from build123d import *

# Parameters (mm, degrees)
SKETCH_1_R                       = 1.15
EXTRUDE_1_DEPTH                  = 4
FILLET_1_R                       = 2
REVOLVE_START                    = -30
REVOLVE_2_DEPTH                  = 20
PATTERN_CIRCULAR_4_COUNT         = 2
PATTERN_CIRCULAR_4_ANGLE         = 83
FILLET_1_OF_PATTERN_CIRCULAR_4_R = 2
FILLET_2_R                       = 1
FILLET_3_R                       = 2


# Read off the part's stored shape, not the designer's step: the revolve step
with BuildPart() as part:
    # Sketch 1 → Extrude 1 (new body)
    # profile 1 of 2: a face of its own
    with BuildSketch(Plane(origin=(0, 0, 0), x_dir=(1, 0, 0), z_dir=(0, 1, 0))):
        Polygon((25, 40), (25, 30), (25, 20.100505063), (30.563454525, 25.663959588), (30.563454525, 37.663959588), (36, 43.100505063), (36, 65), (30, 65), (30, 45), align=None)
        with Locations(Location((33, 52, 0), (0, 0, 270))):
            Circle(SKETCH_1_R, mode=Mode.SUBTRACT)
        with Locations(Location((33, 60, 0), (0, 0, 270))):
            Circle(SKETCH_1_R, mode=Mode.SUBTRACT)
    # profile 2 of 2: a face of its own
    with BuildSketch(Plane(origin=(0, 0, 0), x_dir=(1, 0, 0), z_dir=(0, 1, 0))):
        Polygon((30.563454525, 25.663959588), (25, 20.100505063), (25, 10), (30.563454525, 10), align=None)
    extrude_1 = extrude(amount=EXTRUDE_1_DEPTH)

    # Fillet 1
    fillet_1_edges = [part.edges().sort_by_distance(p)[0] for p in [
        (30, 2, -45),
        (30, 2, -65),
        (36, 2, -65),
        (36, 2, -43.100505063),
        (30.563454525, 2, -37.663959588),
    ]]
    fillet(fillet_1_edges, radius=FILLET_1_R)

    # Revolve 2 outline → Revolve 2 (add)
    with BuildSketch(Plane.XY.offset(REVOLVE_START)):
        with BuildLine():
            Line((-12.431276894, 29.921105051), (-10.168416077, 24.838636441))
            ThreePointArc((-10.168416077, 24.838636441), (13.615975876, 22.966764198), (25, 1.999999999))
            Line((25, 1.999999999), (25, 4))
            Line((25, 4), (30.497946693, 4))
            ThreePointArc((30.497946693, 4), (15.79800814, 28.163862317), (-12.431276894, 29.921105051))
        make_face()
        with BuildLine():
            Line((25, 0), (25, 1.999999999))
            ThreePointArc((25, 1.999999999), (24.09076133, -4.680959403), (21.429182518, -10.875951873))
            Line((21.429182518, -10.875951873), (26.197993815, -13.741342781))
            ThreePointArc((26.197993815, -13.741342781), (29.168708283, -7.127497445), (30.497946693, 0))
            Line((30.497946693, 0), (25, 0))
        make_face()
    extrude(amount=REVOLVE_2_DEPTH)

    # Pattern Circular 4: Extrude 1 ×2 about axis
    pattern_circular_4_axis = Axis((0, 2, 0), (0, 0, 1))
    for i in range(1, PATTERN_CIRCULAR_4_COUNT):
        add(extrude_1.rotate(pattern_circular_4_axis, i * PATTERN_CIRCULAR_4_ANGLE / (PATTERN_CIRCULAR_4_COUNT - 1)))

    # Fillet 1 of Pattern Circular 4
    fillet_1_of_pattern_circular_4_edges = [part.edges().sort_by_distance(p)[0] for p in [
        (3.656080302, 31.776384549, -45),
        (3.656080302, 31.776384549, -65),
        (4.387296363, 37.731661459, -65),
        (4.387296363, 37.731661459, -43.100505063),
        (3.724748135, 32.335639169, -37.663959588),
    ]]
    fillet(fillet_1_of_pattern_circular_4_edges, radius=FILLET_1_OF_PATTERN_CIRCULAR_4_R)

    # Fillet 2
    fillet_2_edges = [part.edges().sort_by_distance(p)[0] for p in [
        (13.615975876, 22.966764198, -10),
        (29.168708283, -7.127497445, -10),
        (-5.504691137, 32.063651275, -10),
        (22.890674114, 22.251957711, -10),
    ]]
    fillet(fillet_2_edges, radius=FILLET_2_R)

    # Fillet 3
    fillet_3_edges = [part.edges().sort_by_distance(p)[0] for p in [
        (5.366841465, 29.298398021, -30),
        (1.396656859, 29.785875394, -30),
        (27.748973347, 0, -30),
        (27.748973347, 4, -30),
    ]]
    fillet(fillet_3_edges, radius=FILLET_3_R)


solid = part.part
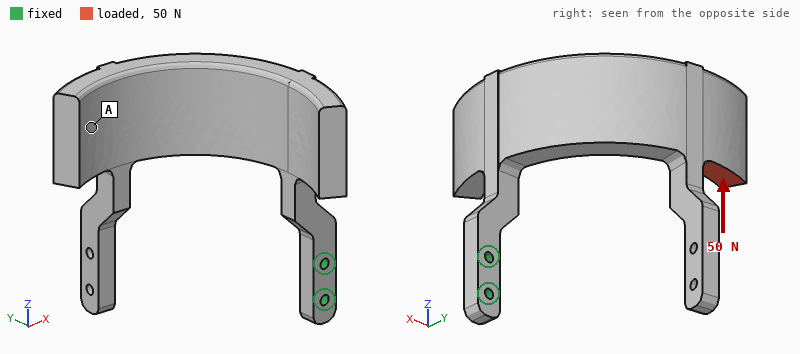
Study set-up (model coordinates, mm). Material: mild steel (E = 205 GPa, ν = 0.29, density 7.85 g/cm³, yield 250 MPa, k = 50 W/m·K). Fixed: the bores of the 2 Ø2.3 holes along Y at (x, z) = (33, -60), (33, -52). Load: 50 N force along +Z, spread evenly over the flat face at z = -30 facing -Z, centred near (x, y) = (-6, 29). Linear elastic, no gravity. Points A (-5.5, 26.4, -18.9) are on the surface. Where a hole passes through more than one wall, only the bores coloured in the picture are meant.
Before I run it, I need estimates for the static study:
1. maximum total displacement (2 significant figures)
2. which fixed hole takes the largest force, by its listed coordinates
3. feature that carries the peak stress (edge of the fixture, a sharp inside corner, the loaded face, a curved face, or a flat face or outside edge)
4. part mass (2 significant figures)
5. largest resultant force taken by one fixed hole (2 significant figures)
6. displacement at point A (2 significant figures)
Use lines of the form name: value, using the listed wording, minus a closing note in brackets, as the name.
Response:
maximum total displacement: 0.37 mm
which fixed hole takes the largest force, by its listed coordinates: (33, -52)
feature that carries the peak stress: a curved face
part mass: 74 g
largest resultant force taken by one fixed hole: 100 N
displacement at point A: 0.30 mm
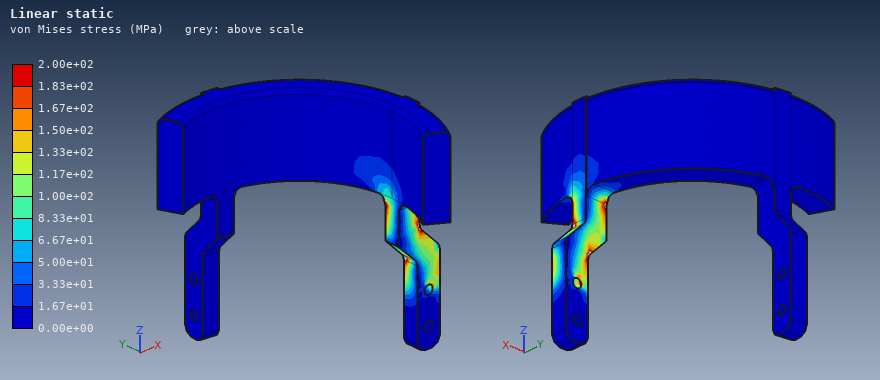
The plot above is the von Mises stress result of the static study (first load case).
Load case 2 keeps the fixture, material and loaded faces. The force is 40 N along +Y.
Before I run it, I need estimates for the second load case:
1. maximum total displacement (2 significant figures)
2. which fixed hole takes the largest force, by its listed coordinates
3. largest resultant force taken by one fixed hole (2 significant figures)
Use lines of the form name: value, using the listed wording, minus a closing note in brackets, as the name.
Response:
maximum total displacement: 0.36 mm
which fixed hole takes the largest force, by its listed coordinates: (33, -52)
largest resultant force taken by one fixed hole: 52 N
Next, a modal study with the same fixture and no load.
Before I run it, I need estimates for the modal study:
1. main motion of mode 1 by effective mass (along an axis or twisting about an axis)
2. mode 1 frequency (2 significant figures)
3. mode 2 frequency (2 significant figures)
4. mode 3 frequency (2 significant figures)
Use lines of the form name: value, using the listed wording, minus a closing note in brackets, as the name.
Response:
main motion of mode 1 by effective mass: along Y
mode 1 frequency: 290 Hz
mode 2 frequency: 330 Hz
mode 3 frequency: 690 Hz
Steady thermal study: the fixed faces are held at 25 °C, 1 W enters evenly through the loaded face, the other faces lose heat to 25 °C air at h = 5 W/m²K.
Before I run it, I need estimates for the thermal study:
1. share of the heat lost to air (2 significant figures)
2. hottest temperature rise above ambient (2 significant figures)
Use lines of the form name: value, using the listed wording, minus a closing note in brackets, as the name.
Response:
share of the heat lost to air: 38 %
hottest temperature rise above ambient: 22 K
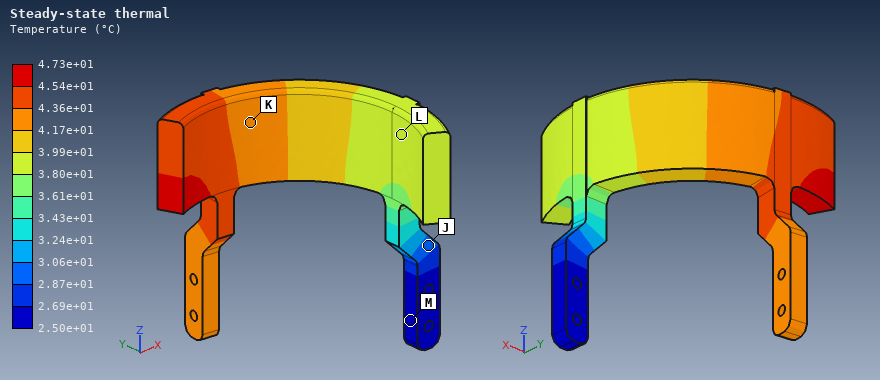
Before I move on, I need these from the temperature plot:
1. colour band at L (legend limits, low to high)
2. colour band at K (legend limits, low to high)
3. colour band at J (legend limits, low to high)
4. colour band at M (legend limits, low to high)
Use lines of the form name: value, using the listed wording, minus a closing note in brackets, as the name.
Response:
colour band at L: 3.80e+01 to 3.99e+01 °C
colour band at K: 4.17e+01 to 4.36e+01 °C
colour band at J: 2.87e+01 to 3.06e+01 °C
colour band at M: 2.50e+01 to 2.69e+01 °C
